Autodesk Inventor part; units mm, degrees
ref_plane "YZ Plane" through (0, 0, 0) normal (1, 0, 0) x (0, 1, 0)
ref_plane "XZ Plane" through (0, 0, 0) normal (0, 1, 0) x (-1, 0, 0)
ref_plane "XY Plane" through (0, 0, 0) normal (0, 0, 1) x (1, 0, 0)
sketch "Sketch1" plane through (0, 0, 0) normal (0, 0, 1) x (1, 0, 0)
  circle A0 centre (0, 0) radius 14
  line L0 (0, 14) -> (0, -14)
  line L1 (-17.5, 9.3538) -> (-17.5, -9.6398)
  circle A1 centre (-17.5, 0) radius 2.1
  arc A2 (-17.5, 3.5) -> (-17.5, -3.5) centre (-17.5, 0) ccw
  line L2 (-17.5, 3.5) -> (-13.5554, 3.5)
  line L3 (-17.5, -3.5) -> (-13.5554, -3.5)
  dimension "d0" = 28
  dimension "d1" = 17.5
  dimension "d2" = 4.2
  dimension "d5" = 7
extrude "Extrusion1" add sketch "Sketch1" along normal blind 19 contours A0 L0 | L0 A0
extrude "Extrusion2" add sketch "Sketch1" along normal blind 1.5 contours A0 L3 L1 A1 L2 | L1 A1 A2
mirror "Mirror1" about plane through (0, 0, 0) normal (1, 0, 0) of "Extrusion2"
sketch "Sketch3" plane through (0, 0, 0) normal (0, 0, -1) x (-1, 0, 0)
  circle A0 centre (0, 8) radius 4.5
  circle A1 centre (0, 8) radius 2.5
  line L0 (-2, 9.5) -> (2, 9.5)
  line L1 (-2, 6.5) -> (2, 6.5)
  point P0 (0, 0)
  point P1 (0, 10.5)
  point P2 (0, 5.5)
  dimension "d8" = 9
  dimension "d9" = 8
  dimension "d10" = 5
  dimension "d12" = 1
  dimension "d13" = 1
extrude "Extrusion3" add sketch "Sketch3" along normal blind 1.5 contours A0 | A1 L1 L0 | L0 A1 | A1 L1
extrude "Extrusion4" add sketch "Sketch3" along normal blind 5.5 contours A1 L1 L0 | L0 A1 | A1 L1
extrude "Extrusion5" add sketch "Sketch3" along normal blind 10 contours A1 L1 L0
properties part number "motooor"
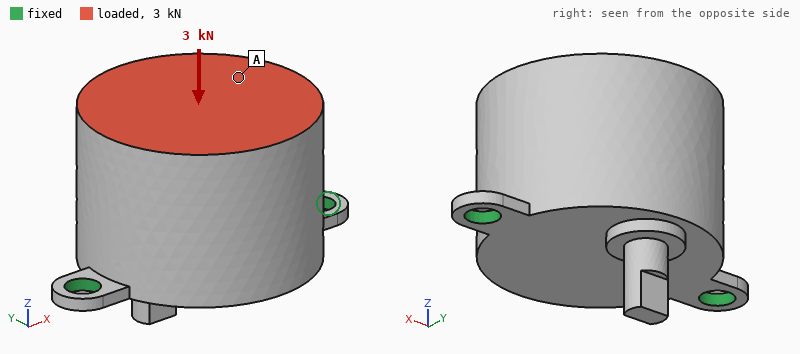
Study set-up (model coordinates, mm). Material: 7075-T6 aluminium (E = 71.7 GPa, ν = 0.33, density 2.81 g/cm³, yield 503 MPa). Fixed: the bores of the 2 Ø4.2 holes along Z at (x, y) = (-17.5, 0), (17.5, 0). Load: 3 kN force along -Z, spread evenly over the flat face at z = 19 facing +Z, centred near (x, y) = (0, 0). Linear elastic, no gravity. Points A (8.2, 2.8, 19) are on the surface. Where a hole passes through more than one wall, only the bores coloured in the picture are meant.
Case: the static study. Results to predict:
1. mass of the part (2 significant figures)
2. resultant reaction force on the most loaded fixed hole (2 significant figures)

34 g
1.7 kN
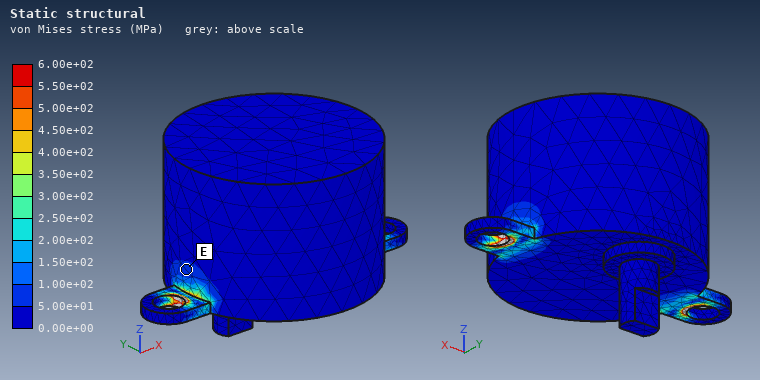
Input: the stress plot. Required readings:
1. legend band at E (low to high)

5.00e+01 to 1.00e+02 MPa
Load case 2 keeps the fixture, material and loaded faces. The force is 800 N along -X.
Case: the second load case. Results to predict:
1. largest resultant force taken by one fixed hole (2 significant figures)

640 N
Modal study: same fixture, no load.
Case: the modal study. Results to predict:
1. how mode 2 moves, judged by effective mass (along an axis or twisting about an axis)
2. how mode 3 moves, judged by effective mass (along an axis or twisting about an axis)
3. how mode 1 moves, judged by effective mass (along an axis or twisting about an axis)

along Z
along X
along Y
